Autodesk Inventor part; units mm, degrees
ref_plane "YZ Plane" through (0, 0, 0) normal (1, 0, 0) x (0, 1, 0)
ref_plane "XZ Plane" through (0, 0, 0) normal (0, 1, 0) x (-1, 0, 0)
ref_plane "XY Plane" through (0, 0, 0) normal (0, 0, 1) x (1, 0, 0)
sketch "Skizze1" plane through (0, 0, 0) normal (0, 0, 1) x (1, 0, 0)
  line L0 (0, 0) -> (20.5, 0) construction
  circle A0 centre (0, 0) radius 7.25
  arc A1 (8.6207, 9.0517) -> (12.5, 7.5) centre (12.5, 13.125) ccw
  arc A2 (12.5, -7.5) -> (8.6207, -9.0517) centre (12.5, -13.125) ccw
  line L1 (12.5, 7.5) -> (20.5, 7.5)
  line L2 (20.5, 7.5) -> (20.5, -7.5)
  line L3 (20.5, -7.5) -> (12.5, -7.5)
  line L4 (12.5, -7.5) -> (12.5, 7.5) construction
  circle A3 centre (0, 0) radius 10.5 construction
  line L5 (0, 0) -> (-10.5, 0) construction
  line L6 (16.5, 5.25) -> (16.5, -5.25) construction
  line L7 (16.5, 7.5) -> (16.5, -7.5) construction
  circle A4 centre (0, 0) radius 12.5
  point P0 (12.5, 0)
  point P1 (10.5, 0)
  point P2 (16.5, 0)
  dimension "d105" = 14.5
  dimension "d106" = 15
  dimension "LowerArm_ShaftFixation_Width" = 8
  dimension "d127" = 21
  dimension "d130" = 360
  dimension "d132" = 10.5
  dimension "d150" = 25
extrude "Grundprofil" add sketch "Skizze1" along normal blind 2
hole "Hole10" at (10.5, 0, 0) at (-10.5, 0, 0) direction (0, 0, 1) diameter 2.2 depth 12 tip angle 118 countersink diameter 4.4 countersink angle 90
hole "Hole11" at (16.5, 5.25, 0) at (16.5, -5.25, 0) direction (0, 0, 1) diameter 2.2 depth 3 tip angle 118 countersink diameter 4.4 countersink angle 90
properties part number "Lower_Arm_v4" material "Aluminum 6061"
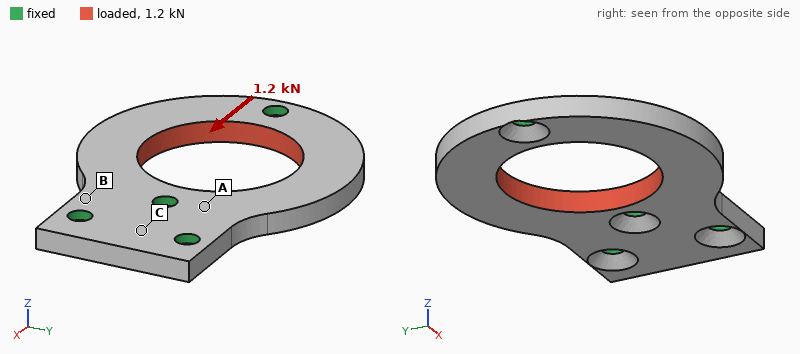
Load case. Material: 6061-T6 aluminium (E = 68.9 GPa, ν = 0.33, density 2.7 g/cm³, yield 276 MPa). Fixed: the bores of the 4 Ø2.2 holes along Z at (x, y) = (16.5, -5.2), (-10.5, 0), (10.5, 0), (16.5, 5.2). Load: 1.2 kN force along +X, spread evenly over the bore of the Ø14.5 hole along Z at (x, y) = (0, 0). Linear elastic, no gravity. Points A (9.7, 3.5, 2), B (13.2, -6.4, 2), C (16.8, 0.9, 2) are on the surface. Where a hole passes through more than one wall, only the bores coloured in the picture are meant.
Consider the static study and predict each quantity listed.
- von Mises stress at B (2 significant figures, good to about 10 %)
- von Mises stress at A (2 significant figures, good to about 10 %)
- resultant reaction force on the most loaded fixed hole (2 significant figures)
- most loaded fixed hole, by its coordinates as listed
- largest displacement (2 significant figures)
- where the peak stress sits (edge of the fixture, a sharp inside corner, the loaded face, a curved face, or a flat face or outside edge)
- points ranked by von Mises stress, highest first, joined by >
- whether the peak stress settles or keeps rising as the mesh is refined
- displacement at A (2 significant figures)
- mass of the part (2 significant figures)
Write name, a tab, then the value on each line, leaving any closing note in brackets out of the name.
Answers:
von Mises stress at B	44 MPa
von Mises stress at A	23 MPa
resultant reaction force on the most loaded fixed hole	460 N
most loaded fixed hole, by its coordinates as listed	(-10.5, 0)
largest displacement	9.1 µm
where the peak stress sits	edge of the fixture
points ranked by von Mises stress, highest first, joined by >	B > A > C
whether the peak stress settles or keeps rising as the mesh is refined	keeps rising
displacement at A	2.0 µm
mass of the part	2.3 g
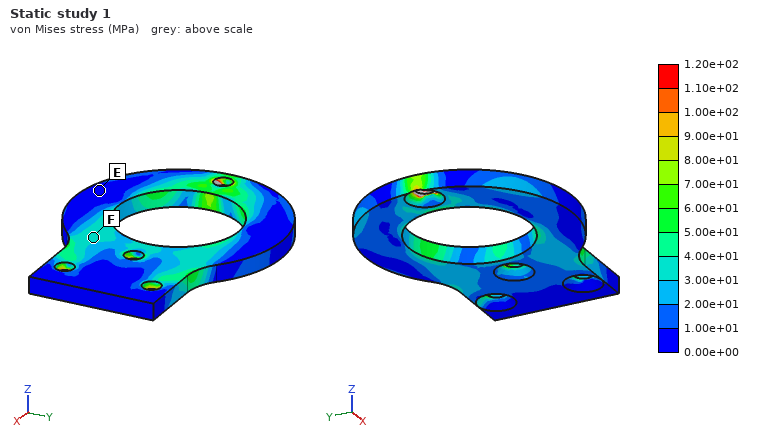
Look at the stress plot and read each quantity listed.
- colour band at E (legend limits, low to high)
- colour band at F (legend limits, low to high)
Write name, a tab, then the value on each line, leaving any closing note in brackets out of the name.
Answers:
colour band at E	0.00e+00 to 1.00e+01 MPa
colour band at F	3.00e+01 to 4.00e+01 MPa
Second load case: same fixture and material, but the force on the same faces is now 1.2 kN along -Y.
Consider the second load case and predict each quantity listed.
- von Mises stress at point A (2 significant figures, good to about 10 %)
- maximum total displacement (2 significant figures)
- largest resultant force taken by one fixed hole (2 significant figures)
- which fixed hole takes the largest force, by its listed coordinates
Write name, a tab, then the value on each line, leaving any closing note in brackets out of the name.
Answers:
von Mises stress at point A	31 MPa
maximum total displacement	23 µm
largest resultant force taken by one fixed hole	600 N
which fixed hole takes the largest force, by its listed coordinates	(-10.5, 0)
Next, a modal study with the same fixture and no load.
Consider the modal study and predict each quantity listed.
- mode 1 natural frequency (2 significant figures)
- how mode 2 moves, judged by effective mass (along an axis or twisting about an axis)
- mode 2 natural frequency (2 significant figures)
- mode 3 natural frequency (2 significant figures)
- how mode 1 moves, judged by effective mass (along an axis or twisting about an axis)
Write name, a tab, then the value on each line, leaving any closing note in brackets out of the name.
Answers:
mode 1 natural frequency	7700 Hz
how mode 2 moves, judged by effective mass	along Z
mode 2 natural frequency	8800 Hz
mode 3 natural frequency	22 kHz
how mode 1 moves, judged by effective mass	twisting about X
